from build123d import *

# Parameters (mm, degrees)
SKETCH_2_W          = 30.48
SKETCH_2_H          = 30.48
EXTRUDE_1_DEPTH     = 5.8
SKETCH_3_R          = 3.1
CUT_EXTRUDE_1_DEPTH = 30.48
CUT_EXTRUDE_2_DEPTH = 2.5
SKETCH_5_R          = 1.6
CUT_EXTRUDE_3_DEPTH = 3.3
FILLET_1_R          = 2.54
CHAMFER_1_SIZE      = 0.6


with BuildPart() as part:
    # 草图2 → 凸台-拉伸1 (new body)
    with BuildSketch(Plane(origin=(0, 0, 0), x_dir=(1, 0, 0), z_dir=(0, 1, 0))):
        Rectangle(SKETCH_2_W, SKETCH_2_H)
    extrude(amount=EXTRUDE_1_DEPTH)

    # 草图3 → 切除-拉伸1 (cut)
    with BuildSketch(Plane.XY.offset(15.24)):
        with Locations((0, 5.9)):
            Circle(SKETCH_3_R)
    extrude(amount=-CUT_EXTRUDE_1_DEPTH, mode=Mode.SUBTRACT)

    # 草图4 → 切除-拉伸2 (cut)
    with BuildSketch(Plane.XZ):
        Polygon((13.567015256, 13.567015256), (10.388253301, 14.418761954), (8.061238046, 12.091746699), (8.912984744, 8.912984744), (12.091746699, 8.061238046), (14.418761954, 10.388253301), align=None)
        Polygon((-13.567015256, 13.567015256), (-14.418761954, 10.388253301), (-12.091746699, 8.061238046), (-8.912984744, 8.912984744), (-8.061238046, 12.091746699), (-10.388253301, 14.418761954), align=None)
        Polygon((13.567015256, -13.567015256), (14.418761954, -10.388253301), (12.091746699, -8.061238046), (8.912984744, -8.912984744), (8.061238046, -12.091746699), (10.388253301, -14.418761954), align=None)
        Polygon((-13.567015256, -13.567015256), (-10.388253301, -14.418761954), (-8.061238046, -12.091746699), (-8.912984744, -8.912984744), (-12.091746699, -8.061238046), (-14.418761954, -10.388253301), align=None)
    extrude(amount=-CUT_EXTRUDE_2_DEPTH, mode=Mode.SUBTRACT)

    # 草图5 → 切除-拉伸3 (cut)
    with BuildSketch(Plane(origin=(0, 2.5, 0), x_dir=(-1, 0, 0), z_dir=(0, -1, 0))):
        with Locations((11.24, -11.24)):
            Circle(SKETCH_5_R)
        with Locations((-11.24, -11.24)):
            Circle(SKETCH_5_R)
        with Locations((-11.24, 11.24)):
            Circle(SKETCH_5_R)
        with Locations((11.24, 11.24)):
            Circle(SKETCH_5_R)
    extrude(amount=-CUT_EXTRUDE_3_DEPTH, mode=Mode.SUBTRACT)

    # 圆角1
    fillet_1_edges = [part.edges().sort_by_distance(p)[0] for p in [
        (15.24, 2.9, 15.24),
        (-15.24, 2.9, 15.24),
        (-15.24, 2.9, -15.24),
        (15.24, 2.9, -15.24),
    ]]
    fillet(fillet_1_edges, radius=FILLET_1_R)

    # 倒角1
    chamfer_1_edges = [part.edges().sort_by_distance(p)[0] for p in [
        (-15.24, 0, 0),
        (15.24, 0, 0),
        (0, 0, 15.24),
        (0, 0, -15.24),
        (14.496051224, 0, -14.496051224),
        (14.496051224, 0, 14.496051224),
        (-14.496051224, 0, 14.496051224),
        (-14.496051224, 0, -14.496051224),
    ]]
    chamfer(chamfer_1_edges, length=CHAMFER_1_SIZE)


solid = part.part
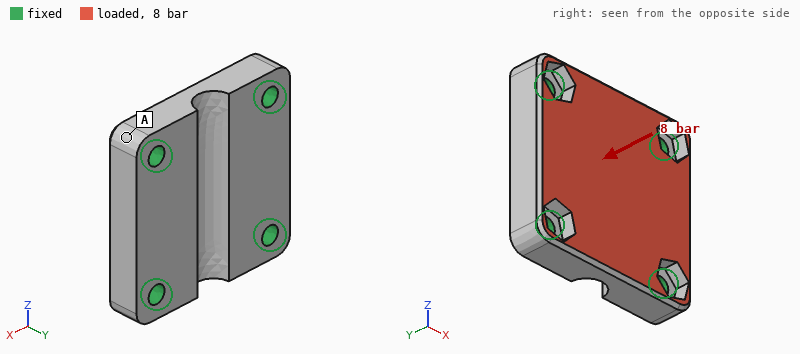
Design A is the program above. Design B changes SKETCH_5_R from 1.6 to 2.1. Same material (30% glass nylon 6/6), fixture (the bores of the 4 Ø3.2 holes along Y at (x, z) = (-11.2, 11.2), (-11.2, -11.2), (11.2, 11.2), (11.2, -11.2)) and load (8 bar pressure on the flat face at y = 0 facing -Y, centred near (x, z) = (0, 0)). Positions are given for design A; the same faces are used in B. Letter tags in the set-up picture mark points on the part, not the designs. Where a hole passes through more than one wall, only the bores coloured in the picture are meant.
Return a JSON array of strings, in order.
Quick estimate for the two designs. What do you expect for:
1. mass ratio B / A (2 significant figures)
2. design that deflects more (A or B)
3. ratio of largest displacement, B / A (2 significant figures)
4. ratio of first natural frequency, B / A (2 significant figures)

["0.98", "A", "0.83", "1.1"]
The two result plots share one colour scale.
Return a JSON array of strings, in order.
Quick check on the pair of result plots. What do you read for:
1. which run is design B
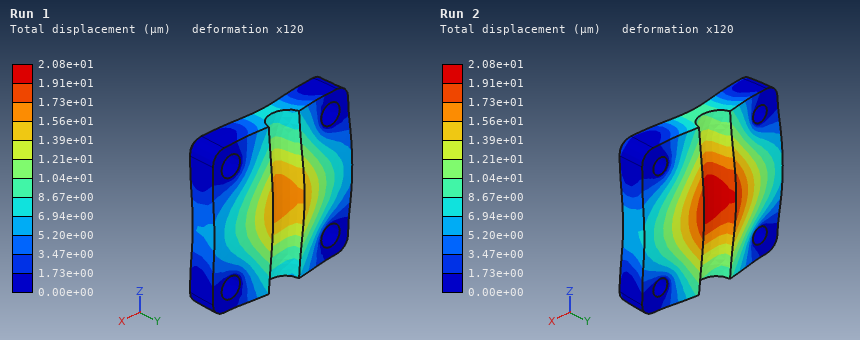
["Run 1"]
